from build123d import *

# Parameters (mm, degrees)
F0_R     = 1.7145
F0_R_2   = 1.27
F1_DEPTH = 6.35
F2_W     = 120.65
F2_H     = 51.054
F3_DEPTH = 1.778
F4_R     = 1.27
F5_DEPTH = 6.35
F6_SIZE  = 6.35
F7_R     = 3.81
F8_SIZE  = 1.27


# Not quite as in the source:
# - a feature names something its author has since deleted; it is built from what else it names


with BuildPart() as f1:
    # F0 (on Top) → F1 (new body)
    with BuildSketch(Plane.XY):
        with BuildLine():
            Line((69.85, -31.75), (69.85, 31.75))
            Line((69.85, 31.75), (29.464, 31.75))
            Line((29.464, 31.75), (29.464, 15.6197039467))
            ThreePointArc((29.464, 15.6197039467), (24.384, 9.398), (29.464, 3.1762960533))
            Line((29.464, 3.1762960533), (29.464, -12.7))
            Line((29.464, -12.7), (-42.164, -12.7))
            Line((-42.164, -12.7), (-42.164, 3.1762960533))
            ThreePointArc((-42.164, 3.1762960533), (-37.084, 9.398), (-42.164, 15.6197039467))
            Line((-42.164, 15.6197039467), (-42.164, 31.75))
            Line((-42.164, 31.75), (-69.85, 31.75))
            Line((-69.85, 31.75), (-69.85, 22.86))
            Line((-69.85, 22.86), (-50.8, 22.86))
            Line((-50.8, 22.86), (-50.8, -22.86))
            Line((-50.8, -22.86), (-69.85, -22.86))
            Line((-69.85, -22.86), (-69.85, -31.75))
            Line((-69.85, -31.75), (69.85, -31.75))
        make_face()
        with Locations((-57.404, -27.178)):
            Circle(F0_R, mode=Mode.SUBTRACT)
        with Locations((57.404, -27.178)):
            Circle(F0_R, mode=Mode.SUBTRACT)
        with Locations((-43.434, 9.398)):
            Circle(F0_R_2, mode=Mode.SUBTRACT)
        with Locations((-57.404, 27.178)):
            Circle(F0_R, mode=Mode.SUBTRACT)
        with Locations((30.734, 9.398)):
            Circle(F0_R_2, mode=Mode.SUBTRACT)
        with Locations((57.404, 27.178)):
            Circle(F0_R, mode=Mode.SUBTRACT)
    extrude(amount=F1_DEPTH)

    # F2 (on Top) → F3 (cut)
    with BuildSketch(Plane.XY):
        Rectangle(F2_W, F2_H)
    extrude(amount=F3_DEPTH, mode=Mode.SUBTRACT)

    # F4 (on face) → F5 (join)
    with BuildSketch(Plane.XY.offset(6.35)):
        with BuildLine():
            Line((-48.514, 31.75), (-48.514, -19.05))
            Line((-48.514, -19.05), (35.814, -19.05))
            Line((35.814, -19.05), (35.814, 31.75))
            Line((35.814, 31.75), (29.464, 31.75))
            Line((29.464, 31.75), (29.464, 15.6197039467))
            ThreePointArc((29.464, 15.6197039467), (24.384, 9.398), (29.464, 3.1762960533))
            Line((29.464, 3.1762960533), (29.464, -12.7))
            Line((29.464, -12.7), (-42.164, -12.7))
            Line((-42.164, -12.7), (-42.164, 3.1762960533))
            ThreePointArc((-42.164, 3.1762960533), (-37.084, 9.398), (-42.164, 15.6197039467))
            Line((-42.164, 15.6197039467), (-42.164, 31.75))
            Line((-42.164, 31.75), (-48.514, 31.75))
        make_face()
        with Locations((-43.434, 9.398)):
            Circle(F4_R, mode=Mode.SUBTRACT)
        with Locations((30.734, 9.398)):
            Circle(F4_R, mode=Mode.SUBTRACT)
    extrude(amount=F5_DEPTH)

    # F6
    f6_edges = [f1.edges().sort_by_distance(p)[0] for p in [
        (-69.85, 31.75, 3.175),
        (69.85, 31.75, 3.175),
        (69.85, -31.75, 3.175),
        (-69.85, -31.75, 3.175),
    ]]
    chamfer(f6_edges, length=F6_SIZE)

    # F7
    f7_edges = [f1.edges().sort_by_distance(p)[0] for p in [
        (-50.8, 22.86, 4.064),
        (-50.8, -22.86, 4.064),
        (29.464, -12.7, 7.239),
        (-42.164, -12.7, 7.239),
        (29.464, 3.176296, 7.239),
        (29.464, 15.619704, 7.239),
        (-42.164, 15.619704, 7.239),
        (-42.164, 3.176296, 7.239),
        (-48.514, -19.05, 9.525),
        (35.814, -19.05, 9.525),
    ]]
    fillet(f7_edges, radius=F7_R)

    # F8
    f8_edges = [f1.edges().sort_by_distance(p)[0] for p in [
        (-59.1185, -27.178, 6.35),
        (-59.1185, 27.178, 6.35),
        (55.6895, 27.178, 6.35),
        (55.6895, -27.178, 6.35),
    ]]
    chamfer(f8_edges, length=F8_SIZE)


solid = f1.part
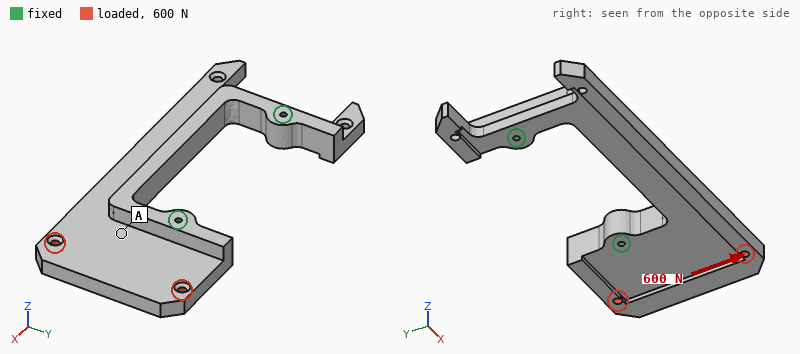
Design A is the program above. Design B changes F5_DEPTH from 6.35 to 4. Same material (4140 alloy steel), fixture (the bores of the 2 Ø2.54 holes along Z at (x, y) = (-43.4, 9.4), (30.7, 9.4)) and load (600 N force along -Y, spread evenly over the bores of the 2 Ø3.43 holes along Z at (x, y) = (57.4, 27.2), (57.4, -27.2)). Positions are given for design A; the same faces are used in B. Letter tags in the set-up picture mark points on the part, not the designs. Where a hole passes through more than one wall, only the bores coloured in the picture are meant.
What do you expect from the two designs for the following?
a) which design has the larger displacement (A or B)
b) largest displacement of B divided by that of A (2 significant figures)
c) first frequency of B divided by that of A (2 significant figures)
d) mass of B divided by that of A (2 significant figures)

B
1.2
0.81
0.91
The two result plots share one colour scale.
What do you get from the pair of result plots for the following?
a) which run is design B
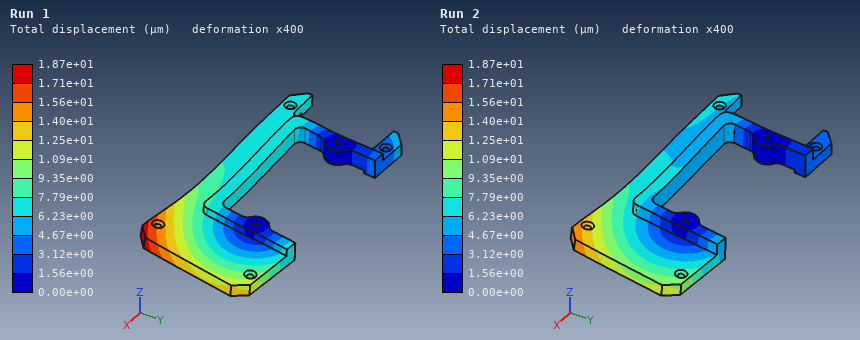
Run 1
